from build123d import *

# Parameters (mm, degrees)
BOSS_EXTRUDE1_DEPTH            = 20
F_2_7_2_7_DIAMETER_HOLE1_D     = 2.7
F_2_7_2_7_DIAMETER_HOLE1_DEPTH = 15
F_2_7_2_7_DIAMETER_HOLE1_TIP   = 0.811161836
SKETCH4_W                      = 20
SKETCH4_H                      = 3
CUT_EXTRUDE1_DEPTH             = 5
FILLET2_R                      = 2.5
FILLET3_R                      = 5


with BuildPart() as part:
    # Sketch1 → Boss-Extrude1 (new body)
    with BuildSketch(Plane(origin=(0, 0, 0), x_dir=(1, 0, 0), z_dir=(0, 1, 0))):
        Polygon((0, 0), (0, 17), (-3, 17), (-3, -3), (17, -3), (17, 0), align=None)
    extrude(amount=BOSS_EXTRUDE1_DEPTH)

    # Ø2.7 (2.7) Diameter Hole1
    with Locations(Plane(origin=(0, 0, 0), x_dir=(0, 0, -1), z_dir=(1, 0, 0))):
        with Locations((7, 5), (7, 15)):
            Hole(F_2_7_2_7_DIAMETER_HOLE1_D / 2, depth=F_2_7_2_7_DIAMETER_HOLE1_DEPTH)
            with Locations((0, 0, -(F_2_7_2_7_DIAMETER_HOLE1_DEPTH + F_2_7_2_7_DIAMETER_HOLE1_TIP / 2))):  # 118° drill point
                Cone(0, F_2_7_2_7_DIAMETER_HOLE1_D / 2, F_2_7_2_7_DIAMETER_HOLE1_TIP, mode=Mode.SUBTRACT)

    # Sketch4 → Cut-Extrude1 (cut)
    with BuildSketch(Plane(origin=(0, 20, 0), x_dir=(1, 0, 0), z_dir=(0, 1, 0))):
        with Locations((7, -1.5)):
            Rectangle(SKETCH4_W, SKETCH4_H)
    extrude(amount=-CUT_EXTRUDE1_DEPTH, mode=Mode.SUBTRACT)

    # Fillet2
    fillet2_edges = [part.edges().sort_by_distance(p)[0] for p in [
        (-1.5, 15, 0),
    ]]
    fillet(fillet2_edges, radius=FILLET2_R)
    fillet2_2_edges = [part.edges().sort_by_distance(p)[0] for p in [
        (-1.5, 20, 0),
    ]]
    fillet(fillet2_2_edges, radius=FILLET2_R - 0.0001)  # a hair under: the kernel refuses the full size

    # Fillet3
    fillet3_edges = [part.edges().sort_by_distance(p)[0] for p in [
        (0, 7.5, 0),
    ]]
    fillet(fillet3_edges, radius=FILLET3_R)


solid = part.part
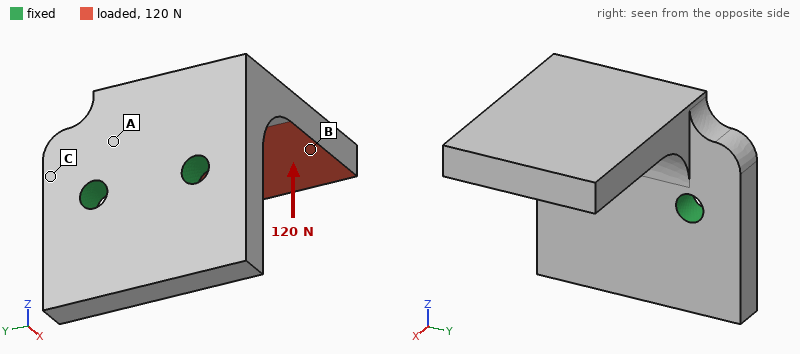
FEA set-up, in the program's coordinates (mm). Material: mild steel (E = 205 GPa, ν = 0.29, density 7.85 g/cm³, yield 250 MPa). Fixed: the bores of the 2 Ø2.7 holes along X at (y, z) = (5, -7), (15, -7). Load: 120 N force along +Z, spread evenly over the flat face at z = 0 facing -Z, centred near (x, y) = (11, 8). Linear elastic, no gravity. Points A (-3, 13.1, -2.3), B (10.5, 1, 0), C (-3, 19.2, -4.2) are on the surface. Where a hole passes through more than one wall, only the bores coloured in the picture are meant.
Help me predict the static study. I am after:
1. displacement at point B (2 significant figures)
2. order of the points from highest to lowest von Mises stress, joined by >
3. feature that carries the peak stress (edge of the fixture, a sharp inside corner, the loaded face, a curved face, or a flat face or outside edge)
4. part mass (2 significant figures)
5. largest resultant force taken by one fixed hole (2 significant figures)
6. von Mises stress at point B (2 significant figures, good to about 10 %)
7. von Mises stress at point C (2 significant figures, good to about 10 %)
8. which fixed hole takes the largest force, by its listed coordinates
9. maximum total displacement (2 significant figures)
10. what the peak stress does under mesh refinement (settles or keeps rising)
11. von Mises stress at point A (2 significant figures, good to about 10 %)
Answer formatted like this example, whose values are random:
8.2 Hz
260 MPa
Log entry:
16 µm
A > C > B
edge of the fixture
15 g
88 N
9.8 MPa
23 MPa
(5, -7)
28 µm
keeps rising
36 MPa
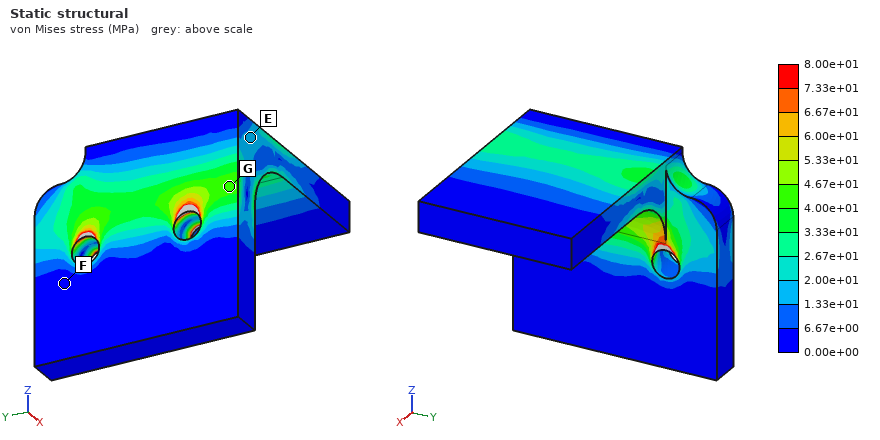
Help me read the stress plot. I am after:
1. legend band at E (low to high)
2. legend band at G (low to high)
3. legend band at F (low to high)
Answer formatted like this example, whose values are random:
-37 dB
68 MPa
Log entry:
1.33e+01 to 2.00e+01 MPa
4.00e+01 to 4.67e+01 MPa
0.00e+00 to 6.67e+00 MPa
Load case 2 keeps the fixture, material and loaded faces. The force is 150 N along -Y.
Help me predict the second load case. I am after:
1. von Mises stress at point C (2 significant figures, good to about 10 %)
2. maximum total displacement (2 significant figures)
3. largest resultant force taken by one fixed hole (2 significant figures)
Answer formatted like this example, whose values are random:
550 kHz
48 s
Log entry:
11 MPa
9.8 µm
190 N
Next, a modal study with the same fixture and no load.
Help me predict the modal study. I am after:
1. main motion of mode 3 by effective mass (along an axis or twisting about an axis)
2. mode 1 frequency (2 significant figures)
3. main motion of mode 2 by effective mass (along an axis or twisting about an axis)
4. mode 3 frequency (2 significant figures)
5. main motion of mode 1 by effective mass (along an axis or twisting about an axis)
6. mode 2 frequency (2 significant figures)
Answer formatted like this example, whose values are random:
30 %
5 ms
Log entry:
along X
5700 Hz
along Y
19 kHz
along Z
12 kHz
